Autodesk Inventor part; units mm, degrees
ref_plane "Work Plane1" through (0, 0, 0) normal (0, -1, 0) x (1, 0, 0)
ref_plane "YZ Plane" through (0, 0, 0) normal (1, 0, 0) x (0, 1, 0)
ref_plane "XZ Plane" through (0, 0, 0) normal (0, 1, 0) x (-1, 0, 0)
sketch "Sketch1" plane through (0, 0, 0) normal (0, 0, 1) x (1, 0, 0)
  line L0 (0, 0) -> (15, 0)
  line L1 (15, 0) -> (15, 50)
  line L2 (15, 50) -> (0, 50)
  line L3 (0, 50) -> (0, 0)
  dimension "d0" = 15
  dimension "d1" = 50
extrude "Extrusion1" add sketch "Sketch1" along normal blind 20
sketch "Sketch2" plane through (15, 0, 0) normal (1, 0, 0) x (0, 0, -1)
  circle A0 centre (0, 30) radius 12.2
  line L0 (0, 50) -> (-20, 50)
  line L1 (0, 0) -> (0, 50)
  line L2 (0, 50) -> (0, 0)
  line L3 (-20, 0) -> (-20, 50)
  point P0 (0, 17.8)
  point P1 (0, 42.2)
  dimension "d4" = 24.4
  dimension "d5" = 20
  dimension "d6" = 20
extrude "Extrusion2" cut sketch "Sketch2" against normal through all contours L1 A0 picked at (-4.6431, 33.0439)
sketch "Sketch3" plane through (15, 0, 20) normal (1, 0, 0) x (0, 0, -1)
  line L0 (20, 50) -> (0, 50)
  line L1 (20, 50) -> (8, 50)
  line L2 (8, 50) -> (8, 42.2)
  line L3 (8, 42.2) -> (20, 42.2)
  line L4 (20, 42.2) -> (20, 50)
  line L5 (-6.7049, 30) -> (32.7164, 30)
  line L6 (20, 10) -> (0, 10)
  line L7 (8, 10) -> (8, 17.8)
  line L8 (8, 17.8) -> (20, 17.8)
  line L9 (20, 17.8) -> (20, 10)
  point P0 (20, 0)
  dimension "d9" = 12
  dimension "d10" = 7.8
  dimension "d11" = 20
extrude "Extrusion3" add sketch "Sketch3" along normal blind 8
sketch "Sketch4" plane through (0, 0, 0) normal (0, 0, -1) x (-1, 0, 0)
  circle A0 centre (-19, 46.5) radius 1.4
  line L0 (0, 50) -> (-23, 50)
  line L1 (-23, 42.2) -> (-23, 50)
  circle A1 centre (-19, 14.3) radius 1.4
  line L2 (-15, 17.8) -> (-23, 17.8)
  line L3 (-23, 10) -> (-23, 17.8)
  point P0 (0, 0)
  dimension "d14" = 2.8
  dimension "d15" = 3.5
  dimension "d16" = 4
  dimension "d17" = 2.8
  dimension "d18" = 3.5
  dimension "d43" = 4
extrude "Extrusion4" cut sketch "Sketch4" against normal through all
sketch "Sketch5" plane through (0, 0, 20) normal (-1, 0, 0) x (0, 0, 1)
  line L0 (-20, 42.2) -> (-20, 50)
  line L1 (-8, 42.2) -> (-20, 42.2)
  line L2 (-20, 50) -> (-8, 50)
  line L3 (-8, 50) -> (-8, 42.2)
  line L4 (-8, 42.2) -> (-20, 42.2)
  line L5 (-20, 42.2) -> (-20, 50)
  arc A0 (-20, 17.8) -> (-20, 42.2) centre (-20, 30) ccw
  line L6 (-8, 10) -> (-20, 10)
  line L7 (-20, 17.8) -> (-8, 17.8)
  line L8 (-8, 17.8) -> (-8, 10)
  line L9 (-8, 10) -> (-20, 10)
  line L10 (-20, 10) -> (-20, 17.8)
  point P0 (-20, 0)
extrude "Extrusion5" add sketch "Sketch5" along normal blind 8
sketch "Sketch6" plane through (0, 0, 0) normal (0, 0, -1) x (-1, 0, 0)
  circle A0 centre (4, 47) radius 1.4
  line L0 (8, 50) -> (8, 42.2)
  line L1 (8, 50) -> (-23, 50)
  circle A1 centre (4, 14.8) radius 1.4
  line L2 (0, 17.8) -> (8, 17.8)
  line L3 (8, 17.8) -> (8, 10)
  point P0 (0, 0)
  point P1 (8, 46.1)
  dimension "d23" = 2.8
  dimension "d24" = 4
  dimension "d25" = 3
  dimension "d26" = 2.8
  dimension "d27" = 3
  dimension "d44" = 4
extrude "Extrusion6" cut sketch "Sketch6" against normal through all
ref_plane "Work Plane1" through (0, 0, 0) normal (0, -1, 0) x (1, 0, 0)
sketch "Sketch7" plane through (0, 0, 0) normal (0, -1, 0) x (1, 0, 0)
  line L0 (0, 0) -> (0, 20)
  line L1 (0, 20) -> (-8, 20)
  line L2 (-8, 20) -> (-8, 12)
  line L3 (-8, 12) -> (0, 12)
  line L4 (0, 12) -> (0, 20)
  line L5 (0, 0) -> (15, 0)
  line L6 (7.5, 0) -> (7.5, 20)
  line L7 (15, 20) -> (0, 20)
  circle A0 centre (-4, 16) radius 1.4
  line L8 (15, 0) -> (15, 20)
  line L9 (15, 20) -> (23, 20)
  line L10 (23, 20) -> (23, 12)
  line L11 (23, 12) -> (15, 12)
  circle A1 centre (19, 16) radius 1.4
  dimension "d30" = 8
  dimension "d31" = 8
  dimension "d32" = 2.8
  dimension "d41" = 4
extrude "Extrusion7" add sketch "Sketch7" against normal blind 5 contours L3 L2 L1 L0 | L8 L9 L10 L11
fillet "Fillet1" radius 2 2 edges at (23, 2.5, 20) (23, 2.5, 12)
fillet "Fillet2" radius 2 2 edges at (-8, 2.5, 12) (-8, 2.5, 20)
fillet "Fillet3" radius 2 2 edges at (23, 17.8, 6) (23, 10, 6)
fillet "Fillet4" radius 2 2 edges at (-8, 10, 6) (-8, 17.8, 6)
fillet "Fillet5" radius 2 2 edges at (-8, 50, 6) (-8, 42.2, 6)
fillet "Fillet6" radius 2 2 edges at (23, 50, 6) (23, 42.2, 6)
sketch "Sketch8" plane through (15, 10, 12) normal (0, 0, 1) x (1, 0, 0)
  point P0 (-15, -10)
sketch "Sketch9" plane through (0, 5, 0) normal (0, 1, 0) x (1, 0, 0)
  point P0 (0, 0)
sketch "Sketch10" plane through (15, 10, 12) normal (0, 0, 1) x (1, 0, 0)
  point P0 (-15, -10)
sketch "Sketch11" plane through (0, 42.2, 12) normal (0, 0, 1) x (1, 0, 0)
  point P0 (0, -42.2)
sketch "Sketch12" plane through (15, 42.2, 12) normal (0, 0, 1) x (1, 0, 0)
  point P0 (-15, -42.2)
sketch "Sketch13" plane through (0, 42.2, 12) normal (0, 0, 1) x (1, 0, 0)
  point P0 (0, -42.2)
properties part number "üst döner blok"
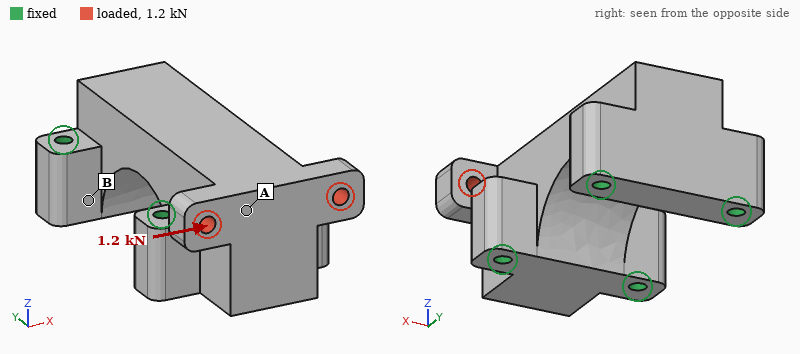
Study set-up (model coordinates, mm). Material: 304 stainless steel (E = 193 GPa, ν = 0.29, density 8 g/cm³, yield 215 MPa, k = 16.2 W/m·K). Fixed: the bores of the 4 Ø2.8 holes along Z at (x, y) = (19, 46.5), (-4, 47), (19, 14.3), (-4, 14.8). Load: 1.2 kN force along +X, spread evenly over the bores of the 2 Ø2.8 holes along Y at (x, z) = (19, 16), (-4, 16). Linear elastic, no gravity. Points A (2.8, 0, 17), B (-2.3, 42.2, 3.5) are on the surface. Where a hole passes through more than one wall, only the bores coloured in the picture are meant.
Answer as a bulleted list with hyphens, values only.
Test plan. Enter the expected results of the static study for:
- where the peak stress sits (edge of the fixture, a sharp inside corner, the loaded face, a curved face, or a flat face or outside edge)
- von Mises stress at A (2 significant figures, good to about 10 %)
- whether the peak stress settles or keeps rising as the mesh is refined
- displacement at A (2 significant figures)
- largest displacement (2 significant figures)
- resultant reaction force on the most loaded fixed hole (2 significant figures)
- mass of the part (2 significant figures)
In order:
- a sharp inside corner
- 15 MPa
- keeps rising
- 3.6 µm
- 5.7 µm
- 990 N
- 120 g
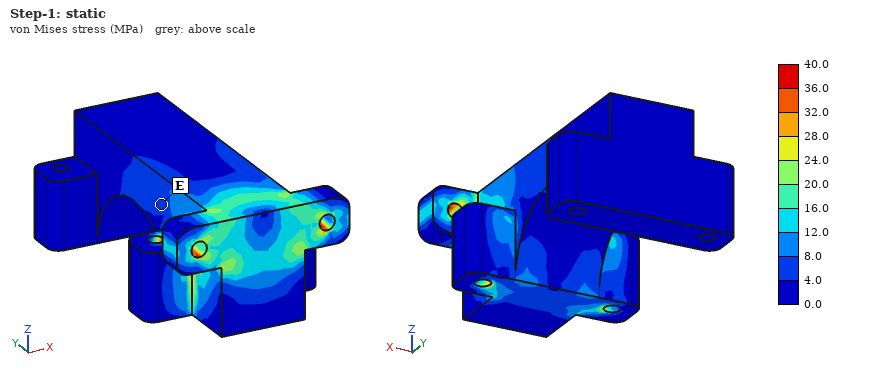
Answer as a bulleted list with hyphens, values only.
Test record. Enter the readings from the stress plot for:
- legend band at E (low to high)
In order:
- 4.0 to 8.0 MPa
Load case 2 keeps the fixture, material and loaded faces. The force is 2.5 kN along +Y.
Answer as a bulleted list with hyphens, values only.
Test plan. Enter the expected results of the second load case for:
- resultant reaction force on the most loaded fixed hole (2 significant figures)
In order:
- 790 N
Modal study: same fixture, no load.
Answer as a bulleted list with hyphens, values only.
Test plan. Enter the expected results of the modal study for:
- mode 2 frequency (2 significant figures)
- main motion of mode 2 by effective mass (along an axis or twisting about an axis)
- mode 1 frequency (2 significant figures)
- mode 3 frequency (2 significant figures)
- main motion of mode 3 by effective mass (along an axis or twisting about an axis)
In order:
- 22 kHz
- along X
- 17 kHz
- 26 kHz
- along Y
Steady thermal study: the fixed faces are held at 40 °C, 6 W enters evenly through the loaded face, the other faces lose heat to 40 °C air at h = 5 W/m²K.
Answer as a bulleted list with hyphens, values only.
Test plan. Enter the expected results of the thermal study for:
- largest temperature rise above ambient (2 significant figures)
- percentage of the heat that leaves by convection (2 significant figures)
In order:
- 62 K
- 4.7 %
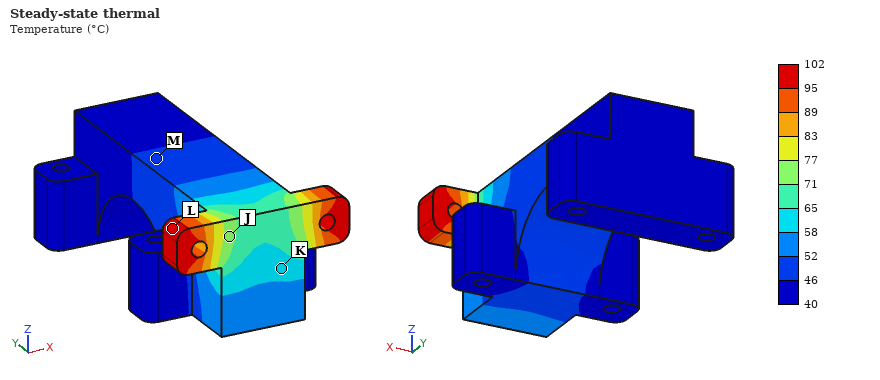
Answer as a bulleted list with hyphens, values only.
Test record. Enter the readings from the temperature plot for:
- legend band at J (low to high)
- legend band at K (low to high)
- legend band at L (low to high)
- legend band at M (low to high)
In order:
- 71 to 77 °C
- 58 to 65 °C
- 95 to 102 °C
- 46 to 52 °C
